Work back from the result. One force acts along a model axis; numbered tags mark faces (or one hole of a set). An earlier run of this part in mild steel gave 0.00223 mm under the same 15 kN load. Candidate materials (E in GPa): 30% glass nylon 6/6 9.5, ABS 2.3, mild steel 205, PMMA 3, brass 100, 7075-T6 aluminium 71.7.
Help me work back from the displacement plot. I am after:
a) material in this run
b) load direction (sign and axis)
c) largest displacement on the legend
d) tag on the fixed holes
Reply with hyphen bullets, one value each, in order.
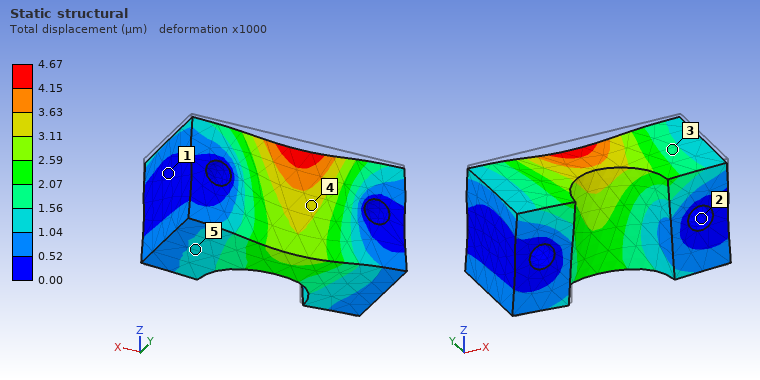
- brass
- -Z
- 4.67 µm
- 2
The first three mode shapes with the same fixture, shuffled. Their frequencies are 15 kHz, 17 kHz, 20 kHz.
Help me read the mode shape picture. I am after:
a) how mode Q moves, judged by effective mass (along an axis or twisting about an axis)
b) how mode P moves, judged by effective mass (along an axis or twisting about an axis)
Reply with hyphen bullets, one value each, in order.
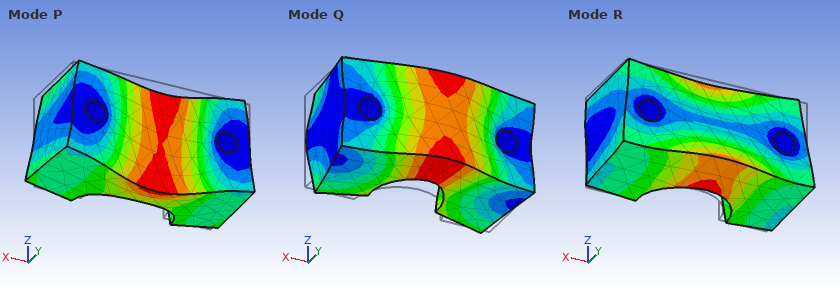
- along Y
- along Z
